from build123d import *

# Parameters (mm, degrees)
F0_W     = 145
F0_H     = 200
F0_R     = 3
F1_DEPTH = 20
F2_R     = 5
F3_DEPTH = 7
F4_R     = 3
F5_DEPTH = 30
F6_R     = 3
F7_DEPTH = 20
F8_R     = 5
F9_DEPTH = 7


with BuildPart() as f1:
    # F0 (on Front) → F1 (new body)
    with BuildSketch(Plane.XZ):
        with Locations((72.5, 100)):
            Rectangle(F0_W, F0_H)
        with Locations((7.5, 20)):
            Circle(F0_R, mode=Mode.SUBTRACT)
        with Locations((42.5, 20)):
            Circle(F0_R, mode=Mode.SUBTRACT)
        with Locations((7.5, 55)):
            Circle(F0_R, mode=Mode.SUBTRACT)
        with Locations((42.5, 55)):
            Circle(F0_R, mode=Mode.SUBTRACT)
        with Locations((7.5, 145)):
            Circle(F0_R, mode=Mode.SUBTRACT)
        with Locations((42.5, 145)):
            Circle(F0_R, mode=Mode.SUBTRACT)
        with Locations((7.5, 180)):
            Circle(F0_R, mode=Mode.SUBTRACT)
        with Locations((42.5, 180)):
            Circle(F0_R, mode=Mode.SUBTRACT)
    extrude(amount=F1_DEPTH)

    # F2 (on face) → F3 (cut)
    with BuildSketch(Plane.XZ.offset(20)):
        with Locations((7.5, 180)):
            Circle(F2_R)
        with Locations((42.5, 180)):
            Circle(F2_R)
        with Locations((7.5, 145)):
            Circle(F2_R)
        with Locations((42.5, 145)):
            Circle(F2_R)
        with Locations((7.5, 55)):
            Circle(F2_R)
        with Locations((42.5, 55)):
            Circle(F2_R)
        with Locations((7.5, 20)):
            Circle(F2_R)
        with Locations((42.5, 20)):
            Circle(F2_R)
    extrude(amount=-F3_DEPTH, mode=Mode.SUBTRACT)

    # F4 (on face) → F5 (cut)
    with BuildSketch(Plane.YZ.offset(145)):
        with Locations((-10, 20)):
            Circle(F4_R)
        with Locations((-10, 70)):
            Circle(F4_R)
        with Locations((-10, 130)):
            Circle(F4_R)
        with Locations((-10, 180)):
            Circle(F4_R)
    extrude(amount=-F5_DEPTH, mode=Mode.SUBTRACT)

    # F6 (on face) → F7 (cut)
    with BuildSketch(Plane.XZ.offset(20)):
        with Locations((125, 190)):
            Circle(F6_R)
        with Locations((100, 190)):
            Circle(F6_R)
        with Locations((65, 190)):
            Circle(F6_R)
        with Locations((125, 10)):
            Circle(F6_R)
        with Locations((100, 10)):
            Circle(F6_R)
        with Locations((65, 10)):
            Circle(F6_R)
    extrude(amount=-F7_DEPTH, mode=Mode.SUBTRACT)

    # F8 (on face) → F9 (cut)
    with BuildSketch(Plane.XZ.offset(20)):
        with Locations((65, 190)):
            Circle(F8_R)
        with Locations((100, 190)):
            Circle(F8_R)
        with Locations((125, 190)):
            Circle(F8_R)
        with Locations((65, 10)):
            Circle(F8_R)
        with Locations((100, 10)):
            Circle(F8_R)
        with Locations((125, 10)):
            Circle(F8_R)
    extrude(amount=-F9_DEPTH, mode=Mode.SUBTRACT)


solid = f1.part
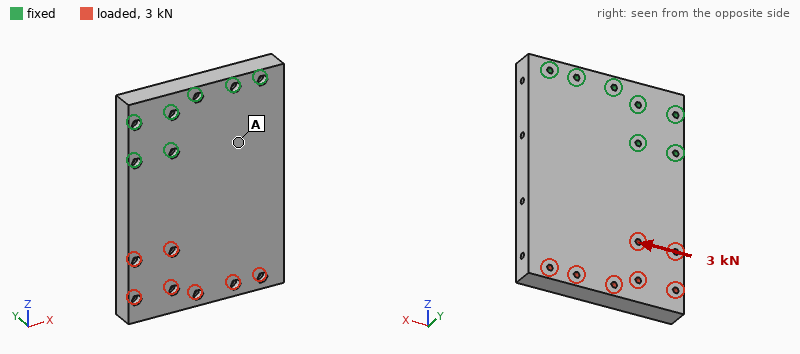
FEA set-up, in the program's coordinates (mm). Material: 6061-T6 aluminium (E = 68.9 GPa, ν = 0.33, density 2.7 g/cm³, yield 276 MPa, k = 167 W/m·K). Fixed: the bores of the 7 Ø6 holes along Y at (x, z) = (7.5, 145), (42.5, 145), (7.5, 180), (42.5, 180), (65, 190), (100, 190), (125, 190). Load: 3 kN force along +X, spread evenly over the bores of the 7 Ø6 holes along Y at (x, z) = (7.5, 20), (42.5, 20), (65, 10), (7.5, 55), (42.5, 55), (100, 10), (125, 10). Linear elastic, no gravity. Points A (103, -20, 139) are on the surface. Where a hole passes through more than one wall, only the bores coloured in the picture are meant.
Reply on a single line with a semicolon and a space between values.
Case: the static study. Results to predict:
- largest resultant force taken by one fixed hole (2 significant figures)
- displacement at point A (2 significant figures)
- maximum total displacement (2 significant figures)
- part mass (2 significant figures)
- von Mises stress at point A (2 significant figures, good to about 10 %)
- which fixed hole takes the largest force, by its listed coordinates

2.6 kN; 4.1 µm; 27 µm; 1.5 kg; 2.3 MPa; (7.5, 145)
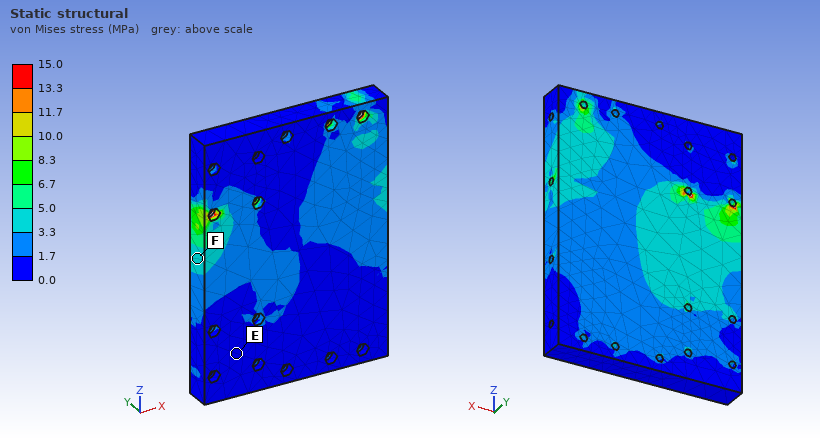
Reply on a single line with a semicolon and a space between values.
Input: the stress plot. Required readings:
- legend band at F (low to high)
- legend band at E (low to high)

3.3 to 5.0 MPa; 0.0 to 1.7 MPa
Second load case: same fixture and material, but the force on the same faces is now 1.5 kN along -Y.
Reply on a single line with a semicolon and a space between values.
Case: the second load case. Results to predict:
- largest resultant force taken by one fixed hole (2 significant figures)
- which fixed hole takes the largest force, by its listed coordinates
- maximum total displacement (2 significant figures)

4.1 kN; (42.5, 145); 0.27 mm
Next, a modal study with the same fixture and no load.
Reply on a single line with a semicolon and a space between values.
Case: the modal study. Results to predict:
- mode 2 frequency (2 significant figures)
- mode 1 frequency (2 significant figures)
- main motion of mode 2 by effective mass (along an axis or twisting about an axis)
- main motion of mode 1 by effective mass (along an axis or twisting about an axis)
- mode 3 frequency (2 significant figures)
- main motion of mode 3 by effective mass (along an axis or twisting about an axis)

1400 Hz; 590 Hz; twisting about Z; along Y; 2800 Hz; along X
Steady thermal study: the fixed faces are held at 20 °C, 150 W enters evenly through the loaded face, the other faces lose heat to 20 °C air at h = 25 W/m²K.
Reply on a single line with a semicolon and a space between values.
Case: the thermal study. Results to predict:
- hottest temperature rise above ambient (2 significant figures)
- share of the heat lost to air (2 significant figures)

41 K; 22 %
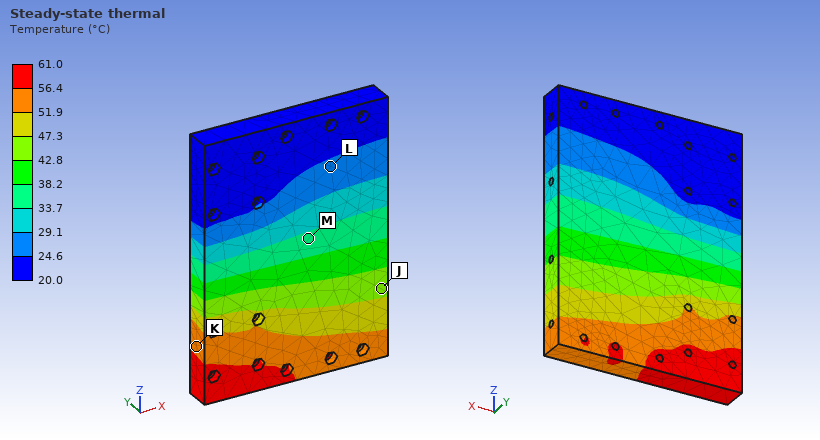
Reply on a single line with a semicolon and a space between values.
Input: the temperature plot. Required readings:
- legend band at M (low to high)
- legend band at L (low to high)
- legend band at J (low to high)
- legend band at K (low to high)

33.7 to 38.2 °C; 24.6 to 29.1 °C; 42.8 to 47.3 °C; 51.9 to 56.4 °C
